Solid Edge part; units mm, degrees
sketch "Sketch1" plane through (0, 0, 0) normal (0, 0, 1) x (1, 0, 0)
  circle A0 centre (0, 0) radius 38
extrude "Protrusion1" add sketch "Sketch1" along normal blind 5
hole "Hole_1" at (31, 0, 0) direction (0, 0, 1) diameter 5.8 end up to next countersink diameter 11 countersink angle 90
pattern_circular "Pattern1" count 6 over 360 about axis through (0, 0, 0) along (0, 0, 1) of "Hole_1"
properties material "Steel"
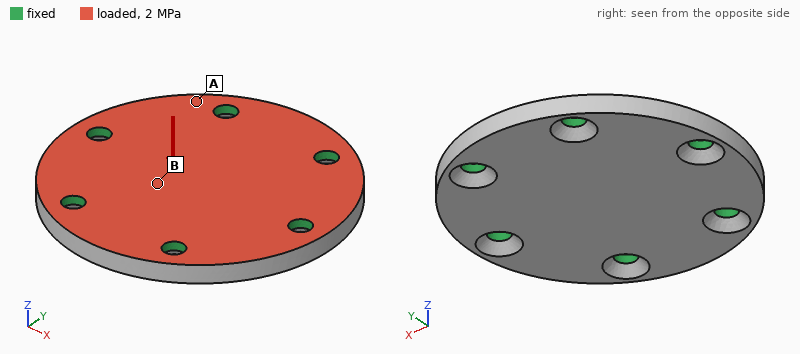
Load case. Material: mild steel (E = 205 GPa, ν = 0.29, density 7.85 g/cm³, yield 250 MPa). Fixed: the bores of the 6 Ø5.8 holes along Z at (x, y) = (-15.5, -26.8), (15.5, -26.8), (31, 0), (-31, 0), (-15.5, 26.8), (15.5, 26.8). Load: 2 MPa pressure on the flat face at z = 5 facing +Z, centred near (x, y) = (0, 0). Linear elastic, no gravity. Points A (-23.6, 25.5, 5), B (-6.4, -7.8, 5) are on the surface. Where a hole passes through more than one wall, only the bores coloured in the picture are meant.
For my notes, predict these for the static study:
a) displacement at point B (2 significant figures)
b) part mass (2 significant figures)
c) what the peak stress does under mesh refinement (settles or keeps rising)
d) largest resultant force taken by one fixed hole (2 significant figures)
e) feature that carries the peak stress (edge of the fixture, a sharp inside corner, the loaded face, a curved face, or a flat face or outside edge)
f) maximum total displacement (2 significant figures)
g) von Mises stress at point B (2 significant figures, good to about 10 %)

16 µm
170 g
keeps rising
1.6 kN
edge of the fixture
19 µm
31 MPa
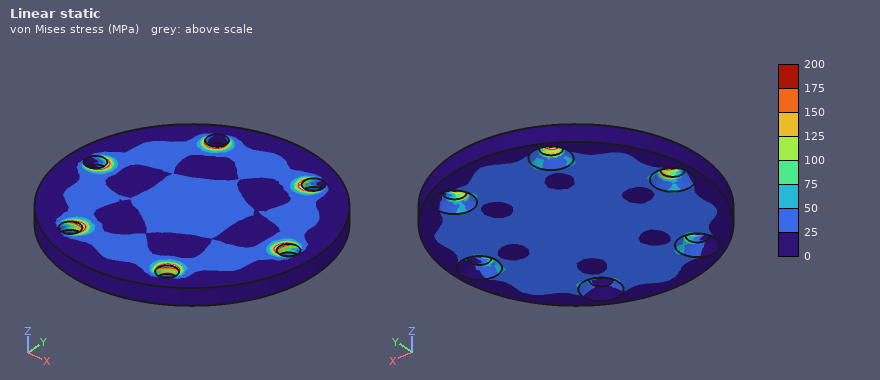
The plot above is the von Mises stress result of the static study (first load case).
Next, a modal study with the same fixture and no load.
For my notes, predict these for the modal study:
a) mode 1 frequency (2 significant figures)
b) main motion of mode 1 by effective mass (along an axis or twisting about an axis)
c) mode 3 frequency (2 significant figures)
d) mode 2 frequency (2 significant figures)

9800 Hz
along Z
18 kHz
18 kHz
